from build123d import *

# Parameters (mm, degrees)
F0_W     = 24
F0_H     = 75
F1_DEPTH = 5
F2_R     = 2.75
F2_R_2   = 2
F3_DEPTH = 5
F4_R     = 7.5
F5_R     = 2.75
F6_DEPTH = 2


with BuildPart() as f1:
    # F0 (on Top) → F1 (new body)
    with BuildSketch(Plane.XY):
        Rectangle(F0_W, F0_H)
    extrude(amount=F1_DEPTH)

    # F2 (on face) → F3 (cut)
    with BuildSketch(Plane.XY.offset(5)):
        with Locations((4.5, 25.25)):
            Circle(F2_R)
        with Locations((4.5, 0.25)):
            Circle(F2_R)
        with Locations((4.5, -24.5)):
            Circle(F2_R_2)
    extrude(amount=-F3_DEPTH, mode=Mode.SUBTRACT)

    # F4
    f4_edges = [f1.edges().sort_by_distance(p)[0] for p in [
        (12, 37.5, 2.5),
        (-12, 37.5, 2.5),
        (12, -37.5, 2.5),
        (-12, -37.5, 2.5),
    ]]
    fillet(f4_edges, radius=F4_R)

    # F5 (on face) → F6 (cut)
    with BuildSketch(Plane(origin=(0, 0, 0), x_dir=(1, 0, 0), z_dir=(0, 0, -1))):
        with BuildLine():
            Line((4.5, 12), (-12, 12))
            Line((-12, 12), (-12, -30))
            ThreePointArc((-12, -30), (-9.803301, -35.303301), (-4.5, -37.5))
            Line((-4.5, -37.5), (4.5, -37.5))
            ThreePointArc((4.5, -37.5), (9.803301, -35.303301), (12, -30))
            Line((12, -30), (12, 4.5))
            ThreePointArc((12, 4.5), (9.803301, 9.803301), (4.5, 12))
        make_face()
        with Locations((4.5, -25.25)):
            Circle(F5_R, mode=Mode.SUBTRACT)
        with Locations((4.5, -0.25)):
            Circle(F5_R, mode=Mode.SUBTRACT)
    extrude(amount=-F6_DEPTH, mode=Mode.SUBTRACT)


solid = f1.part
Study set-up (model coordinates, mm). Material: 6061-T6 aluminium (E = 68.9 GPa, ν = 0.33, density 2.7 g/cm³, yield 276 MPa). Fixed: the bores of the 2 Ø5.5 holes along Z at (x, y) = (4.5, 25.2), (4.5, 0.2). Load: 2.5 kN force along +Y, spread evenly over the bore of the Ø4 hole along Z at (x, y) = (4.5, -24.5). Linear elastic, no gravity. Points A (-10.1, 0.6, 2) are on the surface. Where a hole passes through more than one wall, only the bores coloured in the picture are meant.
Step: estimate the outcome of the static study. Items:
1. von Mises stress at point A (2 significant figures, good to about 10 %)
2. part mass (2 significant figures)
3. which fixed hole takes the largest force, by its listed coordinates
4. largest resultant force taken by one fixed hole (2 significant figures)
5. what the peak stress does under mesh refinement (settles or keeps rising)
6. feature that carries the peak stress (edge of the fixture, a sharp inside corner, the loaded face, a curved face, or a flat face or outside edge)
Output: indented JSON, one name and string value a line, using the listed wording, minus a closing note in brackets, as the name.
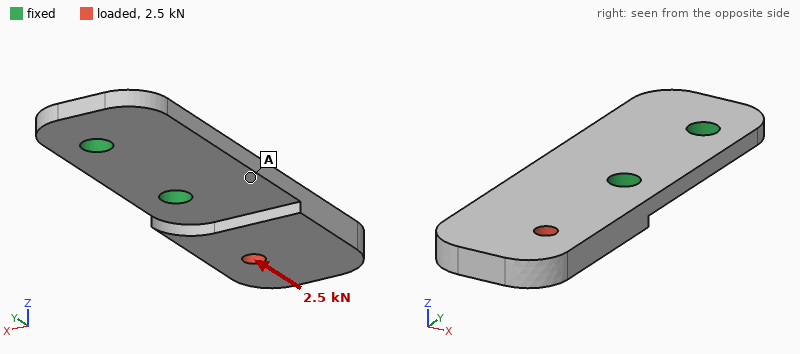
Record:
{
  "von Mises stress at point A": "31 MPa",
  "part mass": "17 g",
  "which fixed hole takes the largest force, by its listed coordinates": "(4.5, 0.2)",
  "largest resultant force taken by one fixed hole": "2.3 kN",
  "what the peak stress does under mesh refinement": "keeps rising",
  "feature that carries the peak stress": "a sharp inside corner"
}
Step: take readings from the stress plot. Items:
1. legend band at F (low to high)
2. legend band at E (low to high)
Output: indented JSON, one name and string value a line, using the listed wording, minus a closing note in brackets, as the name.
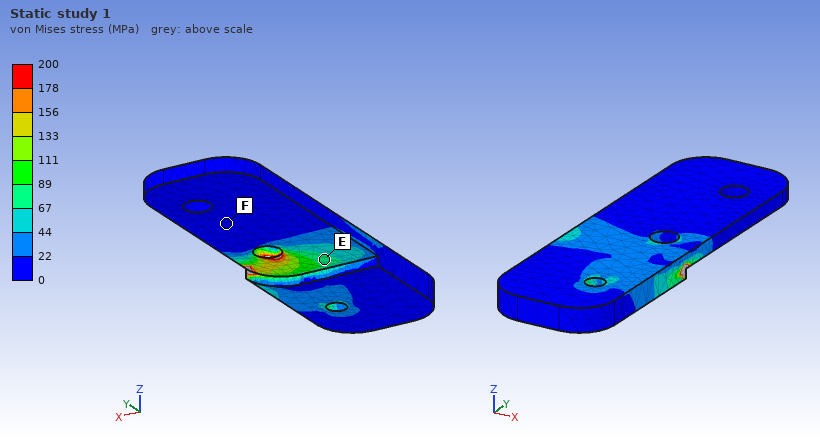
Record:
{
  "legend band at F": "0 to 22 MPa",
  "legend band at E": "67 to 89 MPa"
}
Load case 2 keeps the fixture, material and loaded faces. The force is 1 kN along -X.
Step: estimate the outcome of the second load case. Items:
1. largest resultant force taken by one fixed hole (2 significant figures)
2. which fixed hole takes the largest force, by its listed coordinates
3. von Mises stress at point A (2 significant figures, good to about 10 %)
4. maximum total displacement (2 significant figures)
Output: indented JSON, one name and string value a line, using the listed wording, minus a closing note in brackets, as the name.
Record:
{
  "largest resultant force taken by one fixed hole": "1.7 kN",
  "which fixed hole takes the largest force, by its listed coordinates": "(4.5, 0.2)",
  "von Mises stress at point A": "52 MPa",
  "maximum total displacement": "87 µm"
}
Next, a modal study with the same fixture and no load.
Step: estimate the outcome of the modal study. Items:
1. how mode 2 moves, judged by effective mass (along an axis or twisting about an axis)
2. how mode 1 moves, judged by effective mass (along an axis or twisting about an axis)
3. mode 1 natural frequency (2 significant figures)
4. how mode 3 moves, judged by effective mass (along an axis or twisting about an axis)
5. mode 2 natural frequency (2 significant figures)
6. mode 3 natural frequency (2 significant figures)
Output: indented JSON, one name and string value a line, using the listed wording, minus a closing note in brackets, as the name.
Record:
{
  "how mode 2 moves, judged by effective mass": "twisting about Y",
  "how mode 1 moves, judged by effective mass": "along Z",
  "mode 1 natural frequency": "1600 Hz",
  "how mode 3 moves, judged by effective mass": "along X",
  "mode 2 natural frequency": "5300 Hz",
  "mode 3 natural frequency": "7100 Hz"
}
